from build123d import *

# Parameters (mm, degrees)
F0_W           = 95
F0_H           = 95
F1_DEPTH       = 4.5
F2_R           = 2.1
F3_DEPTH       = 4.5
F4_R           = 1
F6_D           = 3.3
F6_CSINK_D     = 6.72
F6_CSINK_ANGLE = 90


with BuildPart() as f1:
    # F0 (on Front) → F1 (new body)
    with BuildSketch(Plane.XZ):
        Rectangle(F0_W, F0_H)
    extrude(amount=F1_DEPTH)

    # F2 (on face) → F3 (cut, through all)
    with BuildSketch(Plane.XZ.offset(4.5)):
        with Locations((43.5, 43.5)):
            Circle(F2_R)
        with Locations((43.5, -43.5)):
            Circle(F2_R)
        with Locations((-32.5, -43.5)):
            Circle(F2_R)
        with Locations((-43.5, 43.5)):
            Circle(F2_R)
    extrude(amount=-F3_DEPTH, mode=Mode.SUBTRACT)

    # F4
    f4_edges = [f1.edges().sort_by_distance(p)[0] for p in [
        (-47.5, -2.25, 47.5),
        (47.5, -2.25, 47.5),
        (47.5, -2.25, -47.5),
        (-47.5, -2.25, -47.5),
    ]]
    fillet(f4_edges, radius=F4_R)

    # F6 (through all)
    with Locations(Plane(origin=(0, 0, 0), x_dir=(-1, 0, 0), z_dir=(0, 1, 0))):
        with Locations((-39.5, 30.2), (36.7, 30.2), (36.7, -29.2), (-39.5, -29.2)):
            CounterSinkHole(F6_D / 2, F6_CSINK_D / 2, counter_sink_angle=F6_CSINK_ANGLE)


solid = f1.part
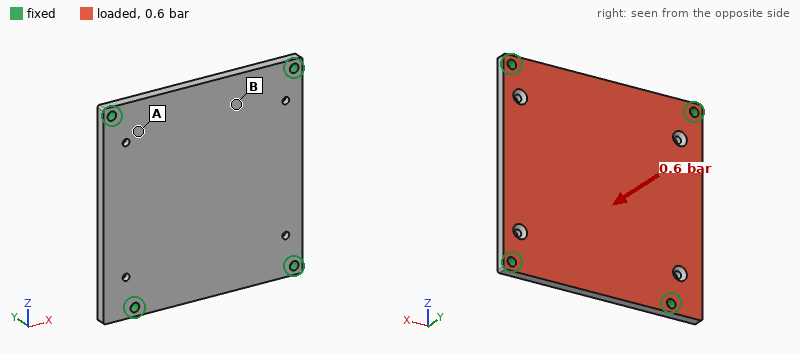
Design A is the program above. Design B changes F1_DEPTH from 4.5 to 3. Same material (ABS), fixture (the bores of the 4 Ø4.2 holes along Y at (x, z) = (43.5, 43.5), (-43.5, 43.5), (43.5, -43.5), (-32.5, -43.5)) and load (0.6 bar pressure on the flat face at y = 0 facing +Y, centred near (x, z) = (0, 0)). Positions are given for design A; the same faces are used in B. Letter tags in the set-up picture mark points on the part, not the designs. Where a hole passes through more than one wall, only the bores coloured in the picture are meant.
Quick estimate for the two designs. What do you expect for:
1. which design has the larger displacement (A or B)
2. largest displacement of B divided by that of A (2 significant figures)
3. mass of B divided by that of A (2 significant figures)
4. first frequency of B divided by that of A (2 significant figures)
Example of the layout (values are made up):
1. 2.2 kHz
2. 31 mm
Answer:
1. B
2. 3.2
3. 0.67
4. 0.69
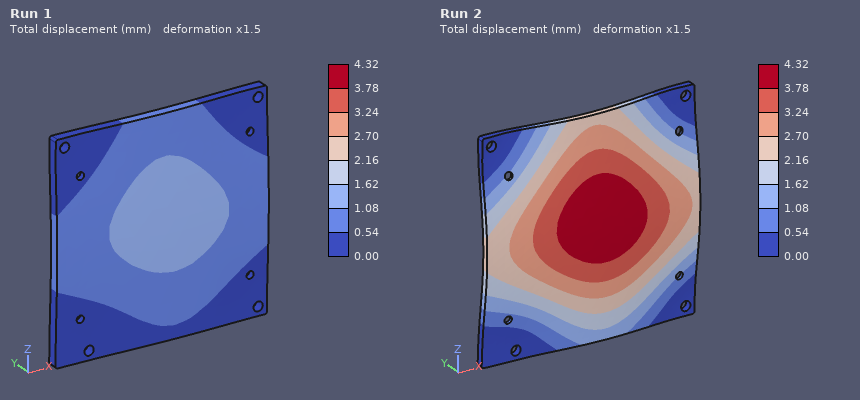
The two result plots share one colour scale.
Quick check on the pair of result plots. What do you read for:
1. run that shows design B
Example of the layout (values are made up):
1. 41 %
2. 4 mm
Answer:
1. Run 2
